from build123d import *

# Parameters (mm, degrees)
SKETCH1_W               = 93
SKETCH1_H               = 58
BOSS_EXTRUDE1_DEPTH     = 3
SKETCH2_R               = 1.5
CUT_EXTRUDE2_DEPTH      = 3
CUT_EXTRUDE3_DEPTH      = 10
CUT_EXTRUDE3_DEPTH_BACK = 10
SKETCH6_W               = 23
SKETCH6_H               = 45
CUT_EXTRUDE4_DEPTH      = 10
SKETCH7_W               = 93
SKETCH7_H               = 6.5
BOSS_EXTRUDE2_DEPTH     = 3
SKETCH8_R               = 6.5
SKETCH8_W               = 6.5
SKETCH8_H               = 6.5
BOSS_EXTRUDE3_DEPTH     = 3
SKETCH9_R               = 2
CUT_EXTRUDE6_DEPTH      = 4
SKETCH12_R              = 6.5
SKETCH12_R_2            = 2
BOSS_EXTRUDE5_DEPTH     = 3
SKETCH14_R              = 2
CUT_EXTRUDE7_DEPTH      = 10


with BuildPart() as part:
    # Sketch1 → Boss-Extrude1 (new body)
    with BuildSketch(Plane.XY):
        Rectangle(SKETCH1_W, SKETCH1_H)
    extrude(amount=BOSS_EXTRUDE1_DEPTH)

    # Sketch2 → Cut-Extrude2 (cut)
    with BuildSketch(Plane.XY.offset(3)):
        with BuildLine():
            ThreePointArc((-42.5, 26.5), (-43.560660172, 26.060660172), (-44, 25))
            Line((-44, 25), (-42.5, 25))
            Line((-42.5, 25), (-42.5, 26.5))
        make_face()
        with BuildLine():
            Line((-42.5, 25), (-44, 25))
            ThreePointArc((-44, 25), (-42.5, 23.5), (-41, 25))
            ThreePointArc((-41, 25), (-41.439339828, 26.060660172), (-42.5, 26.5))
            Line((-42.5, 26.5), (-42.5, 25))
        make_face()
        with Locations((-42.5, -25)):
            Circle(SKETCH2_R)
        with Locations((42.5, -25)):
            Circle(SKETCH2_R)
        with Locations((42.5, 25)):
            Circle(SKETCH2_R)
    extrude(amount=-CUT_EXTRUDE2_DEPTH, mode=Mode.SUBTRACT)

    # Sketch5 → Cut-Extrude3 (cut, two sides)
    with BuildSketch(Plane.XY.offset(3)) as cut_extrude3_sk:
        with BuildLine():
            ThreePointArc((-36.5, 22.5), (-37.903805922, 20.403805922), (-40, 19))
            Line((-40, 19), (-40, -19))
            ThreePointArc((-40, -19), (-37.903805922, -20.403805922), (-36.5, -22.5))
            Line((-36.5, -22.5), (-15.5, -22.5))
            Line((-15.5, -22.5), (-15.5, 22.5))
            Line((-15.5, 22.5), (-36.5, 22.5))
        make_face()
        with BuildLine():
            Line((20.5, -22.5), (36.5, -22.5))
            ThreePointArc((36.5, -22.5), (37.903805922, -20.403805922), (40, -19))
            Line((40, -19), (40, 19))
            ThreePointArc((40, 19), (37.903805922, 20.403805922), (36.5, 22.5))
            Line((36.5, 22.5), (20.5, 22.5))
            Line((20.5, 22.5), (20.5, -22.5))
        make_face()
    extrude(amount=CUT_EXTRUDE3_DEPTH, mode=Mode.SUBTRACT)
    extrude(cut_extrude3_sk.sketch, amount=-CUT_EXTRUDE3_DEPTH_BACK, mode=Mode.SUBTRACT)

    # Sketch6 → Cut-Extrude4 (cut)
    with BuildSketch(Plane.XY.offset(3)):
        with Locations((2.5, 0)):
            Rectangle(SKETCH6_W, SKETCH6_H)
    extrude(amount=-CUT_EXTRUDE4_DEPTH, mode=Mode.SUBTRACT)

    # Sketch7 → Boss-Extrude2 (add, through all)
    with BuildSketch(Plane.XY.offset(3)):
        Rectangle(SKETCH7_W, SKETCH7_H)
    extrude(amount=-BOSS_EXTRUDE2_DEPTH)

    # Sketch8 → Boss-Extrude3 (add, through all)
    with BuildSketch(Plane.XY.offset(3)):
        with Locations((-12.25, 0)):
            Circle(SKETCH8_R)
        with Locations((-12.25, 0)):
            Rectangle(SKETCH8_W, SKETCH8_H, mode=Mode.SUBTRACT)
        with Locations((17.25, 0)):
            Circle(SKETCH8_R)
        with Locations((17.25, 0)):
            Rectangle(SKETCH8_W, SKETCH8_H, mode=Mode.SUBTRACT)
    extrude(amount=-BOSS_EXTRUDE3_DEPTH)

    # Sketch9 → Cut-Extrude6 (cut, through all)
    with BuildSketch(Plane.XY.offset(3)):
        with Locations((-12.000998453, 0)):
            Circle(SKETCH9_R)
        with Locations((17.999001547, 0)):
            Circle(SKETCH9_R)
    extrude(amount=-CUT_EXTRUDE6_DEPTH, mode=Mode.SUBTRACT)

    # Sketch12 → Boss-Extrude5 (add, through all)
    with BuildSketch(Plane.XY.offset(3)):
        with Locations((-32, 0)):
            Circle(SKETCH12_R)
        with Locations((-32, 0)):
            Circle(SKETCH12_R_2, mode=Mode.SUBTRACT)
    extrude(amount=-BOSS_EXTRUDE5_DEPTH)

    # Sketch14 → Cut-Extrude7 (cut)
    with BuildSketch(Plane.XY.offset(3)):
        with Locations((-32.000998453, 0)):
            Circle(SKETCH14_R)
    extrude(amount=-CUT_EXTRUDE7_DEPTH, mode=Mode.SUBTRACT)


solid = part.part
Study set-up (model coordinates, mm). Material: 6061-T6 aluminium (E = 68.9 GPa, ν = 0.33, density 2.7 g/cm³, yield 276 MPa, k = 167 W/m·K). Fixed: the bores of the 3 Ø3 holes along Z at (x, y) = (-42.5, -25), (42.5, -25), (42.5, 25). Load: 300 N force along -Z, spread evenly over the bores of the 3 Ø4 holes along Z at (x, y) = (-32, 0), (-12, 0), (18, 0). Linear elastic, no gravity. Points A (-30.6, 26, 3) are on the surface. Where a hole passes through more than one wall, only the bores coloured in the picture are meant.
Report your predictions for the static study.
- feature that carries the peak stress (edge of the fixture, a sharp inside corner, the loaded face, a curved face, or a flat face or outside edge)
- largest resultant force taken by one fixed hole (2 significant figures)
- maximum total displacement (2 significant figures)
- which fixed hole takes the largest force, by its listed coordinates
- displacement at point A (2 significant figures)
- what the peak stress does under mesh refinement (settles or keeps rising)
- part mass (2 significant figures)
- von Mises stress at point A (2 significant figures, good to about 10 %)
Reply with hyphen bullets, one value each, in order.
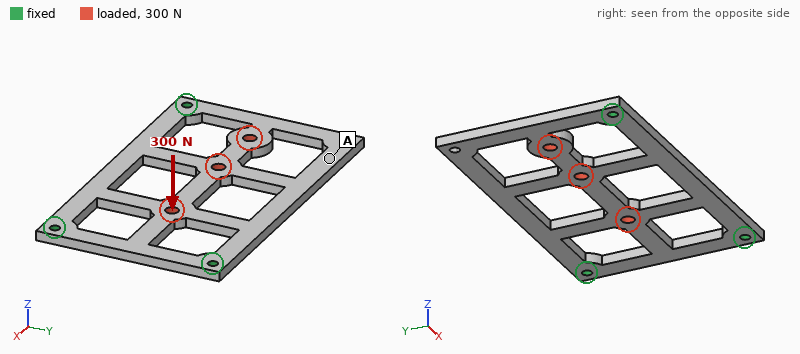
- edge of the fixture
- 160 N
- 0.79 mm
- (-42.5, -25)
- 0.75 mm
- keeps rising
- 23 g
- 49 MPa
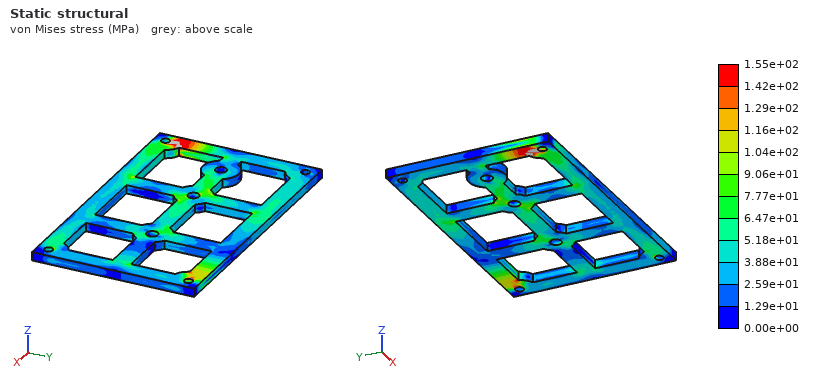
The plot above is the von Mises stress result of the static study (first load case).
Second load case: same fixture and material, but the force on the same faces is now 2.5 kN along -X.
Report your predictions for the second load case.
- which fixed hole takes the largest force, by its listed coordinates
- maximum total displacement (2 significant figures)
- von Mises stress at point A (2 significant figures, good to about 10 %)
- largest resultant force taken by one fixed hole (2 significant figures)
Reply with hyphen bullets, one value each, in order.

- (42.5, 25)
- 0.10 mm
- 22 MPa
- 1.1 kN
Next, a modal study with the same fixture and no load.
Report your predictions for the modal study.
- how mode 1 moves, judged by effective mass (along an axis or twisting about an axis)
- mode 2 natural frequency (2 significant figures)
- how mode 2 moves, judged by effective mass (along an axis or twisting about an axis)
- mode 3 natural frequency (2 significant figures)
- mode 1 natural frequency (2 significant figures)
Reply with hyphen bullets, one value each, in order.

- along Z
- 1700 Hz
- along Z
- 2500 Hz
- 820 Hz
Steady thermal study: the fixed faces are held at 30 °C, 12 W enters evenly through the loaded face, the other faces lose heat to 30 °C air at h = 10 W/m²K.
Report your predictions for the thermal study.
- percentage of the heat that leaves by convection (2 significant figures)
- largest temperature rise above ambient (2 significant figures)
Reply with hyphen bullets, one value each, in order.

- 11 %
- 32 K
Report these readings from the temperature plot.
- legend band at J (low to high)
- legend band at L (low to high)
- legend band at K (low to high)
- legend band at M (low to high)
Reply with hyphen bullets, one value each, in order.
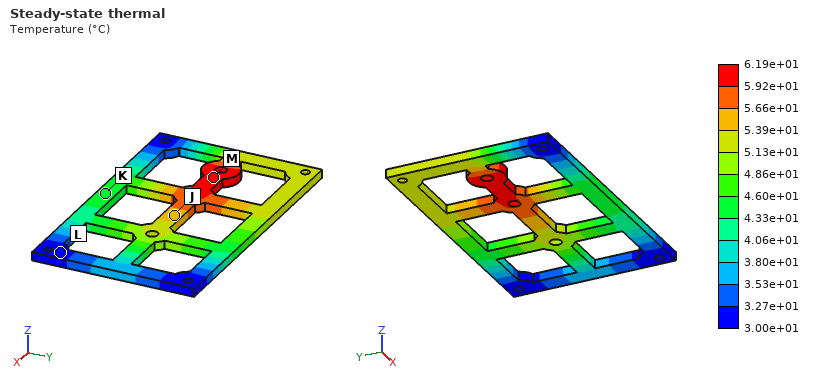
- 5.39e+01 to 5.66e+01 °C
- 3.00e+01 to 3.27e+01 °C
- 4.33e+01 to 4.60e+01 °C
- 5.92e+01 to 6.19e+01 °C
